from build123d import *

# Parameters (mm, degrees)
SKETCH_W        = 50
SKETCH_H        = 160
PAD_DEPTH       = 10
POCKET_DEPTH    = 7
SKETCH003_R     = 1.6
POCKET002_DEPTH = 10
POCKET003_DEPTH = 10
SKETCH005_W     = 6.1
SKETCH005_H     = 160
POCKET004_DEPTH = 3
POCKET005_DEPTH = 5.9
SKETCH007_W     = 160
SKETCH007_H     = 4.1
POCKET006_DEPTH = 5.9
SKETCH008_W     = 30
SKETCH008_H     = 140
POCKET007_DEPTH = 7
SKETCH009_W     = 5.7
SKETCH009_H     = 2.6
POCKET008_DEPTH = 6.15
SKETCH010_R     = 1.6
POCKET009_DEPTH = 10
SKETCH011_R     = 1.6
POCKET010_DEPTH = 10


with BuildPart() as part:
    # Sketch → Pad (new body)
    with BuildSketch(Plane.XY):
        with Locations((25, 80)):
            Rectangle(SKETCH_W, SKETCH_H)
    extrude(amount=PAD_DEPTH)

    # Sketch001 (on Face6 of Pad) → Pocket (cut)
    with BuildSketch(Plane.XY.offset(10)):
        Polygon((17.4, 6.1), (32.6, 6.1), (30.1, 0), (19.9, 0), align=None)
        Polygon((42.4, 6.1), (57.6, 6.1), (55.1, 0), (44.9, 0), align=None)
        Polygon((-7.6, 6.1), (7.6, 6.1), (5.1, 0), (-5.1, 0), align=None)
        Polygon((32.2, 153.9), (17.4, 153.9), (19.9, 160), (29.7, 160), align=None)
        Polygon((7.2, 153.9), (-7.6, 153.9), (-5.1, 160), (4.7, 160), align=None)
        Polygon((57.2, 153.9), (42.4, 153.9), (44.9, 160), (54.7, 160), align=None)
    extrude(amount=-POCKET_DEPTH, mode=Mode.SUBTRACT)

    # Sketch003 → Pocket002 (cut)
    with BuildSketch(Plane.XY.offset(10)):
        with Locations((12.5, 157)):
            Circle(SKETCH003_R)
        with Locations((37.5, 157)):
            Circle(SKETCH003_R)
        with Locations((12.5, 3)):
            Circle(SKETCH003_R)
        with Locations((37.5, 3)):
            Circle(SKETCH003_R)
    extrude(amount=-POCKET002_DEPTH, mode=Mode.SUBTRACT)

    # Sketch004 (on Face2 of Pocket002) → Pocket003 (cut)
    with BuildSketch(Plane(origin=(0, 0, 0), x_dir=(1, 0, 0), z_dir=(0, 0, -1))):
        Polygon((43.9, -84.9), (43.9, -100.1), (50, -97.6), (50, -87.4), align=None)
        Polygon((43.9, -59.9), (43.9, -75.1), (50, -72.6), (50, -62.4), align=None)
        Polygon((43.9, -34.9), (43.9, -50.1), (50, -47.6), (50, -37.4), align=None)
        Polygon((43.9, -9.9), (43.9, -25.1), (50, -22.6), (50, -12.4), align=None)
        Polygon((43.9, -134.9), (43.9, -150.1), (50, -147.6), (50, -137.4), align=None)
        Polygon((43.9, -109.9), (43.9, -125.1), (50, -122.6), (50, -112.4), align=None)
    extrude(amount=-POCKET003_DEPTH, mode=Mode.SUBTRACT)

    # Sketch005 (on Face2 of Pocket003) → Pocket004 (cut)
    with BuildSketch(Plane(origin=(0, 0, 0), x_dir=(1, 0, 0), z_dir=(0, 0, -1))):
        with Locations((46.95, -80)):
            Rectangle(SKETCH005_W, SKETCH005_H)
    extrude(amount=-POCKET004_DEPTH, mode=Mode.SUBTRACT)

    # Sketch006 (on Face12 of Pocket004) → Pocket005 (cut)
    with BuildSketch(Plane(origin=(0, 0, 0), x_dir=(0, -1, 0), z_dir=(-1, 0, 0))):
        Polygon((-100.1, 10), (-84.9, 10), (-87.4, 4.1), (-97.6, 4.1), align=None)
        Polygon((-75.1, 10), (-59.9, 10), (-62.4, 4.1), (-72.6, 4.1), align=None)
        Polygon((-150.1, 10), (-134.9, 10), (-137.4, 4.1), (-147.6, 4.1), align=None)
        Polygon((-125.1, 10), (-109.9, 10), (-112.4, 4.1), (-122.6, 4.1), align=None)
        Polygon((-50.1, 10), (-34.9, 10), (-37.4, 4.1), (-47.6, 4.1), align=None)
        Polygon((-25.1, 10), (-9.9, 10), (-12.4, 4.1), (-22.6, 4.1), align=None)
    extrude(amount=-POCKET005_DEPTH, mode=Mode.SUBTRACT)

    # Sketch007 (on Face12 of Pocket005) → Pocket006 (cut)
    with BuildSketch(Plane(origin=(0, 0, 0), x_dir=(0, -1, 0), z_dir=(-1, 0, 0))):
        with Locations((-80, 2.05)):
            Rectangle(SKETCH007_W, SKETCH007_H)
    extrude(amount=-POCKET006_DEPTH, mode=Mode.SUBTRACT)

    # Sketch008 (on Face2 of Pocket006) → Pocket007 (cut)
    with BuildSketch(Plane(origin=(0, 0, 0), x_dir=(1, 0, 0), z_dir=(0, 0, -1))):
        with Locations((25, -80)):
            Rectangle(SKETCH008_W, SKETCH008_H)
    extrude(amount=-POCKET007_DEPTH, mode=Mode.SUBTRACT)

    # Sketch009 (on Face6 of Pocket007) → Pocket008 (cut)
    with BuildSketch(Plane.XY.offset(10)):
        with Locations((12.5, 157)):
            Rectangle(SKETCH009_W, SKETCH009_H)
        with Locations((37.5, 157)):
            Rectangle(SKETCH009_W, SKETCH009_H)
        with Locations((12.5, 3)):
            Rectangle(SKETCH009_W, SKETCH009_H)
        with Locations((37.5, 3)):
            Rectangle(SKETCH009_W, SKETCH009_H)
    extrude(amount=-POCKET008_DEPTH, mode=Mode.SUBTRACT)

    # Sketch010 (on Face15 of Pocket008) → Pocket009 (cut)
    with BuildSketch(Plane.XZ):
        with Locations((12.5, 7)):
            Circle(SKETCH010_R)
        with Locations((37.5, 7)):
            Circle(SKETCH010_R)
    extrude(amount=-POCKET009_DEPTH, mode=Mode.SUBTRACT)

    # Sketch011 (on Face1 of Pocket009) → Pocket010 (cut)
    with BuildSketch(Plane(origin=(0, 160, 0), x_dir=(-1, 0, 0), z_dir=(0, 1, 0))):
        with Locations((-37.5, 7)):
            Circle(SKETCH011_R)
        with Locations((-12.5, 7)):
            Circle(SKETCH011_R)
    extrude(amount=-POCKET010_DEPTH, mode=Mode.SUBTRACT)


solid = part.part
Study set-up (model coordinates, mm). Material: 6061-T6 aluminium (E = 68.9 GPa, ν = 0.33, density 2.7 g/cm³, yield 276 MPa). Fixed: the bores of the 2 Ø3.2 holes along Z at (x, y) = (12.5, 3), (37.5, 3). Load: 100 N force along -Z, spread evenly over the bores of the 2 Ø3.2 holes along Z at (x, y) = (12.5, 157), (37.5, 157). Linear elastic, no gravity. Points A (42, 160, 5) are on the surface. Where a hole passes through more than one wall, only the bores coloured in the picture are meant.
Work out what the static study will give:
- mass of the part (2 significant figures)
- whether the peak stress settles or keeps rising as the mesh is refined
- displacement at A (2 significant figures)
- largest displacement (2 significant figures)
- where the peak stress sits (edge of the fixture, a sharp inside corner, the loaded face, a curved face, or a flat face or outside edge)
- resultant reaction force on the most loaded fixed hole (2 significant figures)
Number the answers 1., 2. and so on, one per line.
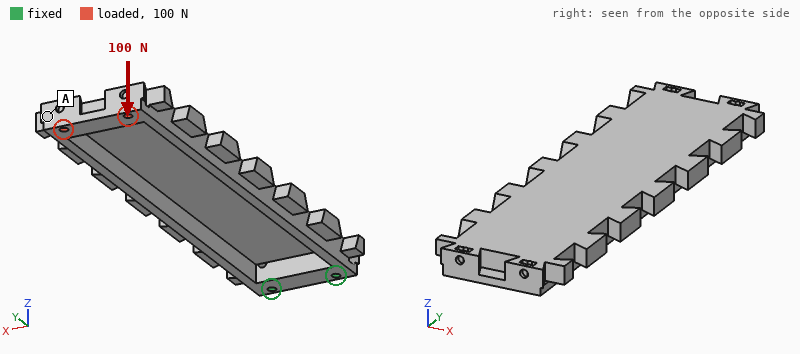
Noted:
1. 95 g
2. keeps rising
3. 1.8 mm
4. 1.8 mm
5. edge of the fixture
6. 330 N
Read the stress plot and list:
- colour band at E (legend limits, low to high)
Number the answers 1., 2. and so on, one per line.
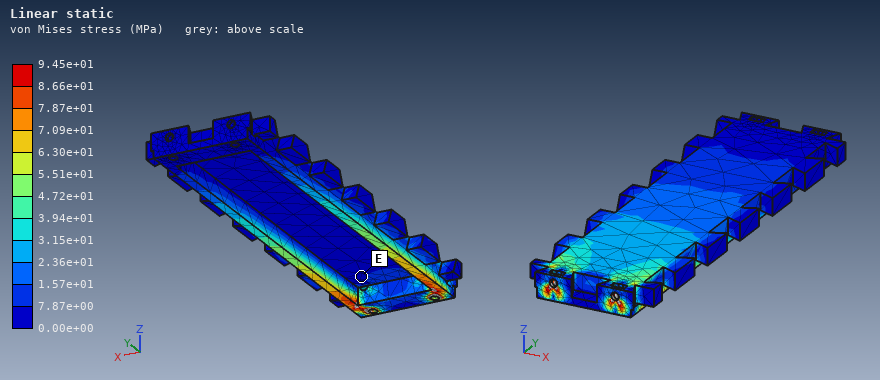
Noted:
1. 0.00e+00 to 7.87e+00 MPa
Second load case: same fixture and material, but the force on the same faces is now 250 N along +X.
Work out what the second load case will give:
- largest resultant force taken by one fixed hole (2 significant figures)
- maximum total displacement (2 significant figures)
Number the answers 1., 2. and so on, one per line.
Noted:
1. 1.4 kN
2. 0.46 mm
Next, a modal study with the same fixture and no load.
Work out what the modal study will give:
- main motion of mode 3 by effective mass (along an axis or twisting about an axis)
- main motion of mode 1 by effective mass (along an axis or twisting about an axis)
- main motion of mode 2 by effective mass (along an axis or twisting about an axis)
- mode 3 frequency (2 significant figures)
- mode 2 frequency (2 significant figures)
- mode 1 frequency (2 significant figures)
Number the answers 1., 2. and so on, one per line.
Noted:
1. along X
2. along Z
3. along X
4. 1200 Hz
5. 670 Hz
6. 240 Hz
